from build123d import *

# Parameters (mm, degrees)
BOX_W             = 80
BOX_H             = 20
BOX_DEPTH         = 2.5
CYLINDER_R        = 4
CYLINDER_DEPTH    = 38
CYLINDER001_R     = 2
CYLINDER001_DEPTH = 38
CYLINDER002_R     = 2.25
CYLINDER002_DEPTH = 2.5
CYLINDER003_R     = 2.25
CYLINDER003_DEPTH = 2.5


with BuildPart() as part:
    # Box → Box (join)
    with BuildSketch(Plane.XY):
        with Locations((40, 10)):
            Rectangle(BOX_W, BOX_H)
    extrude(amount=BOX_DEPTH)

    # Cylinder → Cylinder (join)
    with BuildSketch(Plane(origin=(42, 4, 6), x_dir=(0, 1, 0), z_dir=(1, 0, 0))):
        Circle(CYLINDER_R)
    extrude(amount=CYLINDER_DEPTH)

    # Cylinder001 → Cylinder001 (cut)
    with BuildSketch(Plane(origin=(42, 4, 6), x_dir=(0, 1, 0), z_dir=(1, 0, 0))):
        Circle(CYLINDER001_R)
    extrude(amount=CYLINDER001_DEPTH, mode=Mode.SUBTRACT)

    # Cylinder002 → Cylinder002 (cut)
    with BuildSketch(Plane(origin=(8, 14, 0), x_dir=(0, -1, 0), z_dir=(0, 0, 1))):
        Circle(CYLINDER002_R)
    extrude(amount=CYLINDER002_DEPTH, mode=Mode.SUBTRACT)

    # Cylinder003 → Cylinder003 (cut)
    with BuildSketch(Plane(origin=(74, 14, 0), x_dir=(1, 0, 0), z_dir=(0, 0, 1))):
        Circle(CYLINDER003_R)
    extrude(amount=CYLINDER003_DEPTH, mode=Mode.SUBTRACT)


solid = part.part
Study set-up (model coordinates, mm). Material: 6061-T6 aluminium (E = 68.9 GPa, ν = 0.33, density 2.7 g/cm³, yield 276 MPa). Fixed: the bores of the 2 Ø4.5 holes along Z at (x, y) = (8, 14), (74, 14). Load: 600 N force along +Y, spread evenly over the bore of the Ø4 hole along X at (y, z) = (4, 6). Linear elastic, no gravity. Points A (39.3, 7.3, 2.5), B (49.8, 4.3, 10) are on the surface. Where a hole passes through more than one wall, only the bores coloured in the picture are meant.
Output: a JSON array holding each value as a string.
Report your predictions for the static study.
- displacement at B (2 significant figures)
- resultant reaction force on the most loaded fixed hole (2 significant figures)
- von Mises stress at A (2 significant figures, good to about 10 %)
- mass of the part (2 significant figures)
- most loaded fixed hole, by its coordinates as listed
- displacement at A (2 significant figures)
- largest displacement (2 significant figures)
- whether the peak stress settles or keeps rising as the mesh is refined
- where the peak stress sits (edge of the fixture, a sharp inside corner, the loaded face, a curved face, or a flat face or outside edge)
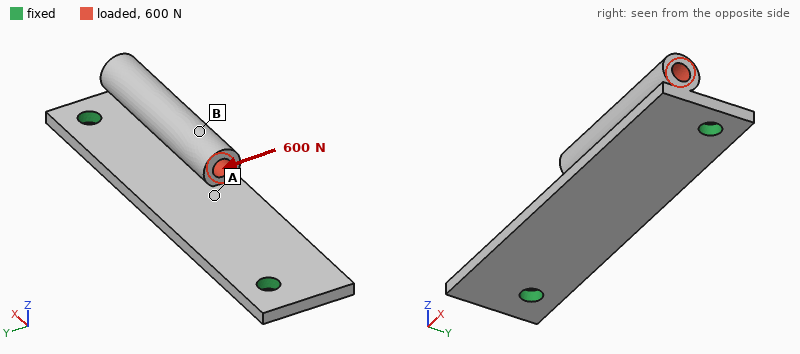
["0.12 mm", "510 N", "32 MPa", "14 g", "(74, 14)", "0.042 mm", "0.13 mm", "keeps rising", "edge of the fixture"]
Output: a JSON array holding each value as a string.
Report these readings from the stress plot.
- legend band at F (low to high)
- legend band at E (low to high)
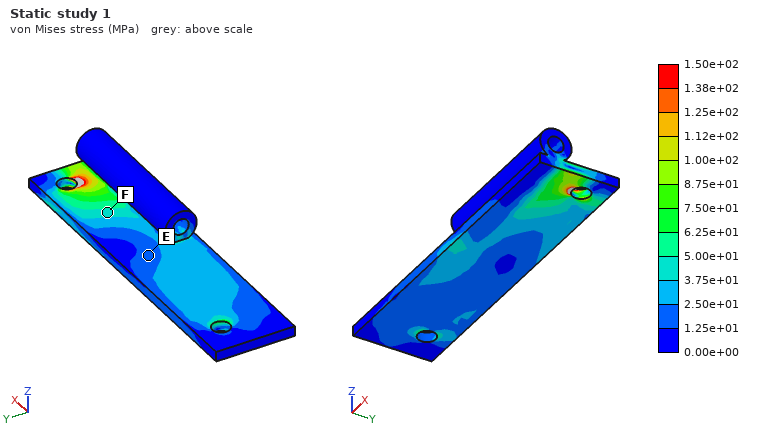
["3.75e+01 to 5.00e+01 MPa", "1.25e+01 to 2.50e+01 MPa"]
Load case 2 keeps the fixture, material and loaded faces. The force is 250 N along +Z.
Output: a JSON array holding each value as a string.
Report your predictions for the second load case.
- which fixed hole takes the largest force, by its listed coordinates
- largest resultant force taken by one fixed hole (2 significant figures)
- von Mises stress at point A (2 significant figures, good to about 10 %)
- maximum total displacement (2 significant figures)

["(74, 14)", "210 N", "34 MPa", "0.13 mm"]
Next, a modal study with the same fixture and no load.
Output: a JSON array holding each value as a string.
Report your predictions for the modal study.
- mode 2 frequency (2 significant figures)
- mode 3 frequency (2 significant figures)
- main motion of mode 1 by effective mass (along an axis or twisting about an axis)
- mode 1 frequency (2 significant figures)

["4700 Hz", "8800 Hz", "along Z", "2700 Hz"]
